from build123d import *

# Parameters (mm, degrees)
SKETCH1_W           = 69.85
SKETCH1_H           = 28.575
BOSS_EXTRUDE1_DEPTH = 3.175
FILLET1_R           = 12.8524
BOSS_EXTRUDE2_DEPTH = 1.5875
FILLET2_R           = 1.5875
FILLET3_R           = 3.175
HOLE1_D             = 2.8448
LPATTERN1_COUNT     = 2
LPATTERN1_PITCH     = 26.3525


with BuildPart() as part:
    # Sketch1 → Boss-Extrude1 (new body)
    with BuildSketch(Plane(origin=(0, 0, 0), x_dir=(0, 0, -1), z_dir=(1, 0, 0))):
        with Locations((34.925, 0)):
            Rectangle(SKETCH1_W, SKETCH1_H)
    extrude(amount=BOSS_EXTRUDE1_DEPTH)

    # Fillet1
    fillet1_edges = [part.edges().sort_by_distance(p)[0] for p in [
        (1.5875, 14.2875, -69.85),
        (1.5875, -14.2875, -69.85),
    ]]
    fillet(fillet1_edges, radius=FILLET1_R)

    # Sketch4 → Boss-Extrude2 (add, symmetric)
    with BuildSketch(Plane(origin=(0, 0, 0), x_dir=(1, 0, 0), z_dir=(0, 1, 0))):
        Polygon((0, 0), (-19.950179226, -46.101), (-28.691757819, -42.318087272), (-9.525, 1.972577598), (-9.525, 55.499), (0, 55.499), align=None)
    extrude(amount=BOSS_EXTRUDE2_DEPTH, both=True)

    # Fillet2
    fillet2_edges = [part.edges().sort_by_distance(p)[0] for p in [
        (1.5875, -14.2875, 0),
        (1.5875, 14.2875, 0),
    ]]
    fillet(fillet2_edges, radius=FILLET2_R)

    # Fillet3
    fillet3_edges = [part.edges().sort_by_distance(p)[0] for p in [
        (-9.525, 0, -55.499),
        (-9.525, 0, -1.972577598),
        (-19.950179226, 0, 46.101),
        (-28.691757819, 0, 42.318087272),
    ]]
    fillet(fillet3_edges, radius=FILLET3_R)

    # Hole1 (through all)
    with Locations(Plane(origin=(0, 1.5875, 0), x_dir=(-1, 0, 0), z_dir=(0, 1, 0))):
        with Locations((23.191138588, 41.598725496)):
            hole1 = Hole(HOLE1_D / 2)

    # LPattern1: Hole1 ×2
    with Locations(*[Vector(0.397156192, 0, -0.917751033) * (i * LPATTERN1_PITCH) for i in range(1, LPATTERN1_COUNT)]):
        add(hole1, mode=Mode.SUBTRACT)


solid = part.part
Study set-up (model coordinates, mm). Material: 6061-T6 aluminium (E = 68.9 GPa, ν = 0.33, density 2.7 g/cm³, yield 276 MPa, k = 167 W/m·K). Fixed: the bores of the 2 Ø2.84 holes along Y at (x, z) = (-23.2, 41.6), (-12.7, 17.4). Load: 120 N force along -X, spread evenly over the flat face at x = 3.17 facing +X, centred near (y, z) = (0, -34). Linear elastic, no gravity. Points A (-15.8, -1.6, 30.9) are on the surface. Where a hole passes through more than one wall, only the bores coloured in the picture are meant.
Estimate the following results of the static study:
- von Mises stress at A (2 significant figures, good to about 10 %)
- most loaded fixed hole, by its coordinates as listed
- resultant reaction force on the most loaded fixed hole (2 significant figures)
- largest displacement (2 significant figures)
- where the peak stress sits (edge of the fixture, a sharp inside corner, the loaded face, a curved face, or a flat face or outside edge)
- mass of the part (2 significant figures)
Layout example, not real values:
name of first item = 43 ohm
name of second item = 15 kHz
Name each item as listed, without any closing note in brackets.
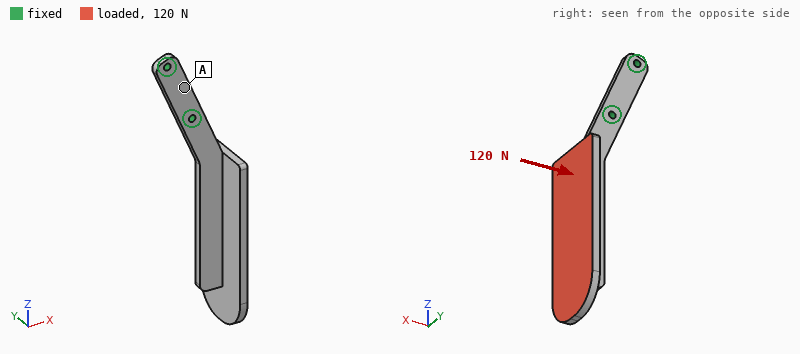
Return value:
von Mises stress at A = 13 MPa
most loaded fixed hole, by its coordinates as listed = (-12.7, 17.4)
resultant reaction force on the most loaded fixed hole = 230 N
largest displacement = 0.74 mm
where the peak stress sits = edge of the fixture
mass of the part = 25 g
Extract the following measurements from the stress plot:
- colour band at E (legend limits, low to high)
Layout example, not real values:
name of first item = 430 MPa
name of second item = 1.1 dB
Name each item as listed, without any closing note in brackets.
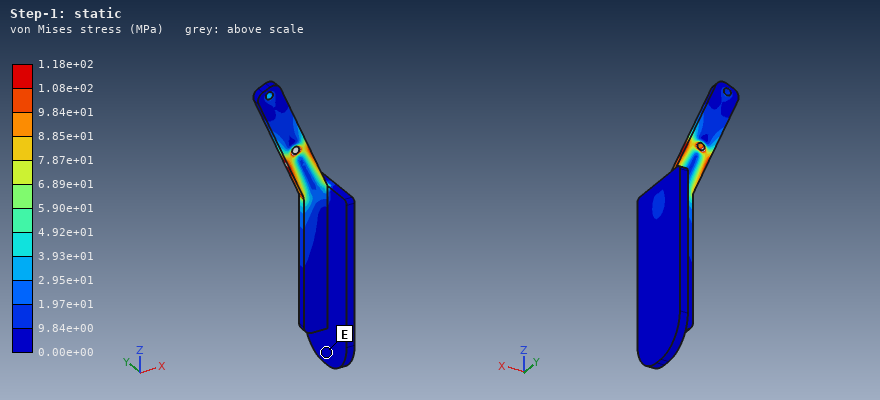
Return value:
colour band at E = 0.00e+00 to 9.84e+00 MPa
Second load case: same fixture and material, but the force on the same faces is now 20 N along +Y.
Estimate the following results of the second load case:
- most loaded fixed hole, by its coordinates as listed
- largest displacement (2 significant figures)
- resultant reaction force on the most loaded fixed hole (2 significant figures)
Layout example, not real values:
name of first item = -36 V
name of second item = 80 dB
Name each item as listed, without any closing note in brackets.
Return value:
most loaded fixed hole, by its coordinates as listed = (-12.7, 17.4)
largest displacement = 0.85 mm
resultant reaction force on the most loaded fixed hole = 22 N
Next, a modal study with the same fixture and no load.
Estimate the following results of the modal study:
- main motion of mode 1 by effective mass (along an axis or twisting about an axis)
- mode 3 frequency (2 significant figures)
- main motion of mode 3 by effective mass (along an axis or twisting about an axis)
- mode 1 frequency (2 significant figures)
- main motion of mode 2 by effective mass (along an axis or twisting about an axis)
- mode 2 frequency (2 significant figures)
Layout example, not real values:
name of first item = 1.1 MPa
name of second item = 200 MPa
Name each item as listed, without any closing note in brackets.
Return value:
main motion of mode 1 by effective mass = along Y
mode 3 frequency = 1200 Hz
main motion of mode 3 by effective mass = twisting about Z
mode 1 frequency = 210 Hz
main motion of mode 2 by effective mass = along X
mode 2 frequency = 560 Hz
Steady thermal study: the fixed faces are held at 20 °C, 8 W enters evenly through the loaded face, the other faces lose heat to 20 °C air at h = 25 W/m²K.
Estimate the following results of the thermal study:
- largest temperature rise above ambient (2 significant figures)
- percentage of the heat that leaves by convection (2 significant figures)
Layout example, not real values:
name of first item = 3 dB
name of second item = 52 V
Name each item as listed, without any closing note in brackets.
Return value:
largest temperature rise above ambient = 34 K
percentage of the heat that leaves by convection = 35 %
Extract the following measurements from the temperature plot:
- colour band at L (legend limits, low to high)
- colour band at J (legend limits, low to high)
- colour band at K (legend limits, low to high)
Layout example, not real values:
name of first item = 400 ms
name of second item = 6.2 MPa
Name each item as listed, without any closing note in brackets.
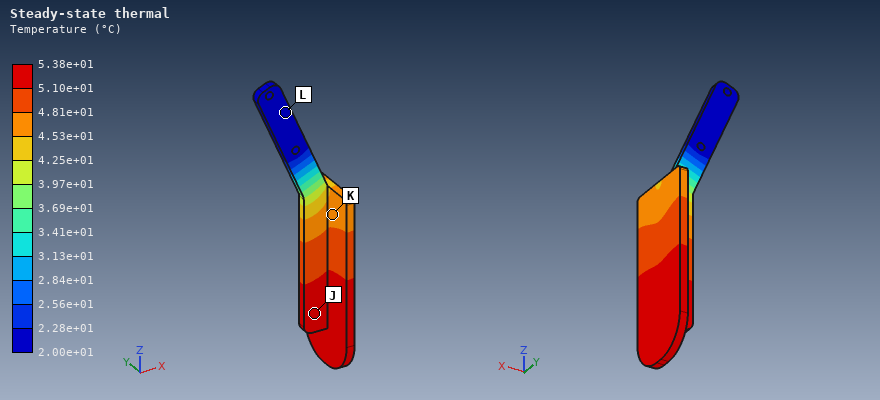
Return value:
colour band at L = 2.00e+01 to 2.28e+01 °C
colour band at J = 5.10e+01 to 5.38e+01 °C
colour band at K = 4.53e+01 to 4.81e+01 °C
